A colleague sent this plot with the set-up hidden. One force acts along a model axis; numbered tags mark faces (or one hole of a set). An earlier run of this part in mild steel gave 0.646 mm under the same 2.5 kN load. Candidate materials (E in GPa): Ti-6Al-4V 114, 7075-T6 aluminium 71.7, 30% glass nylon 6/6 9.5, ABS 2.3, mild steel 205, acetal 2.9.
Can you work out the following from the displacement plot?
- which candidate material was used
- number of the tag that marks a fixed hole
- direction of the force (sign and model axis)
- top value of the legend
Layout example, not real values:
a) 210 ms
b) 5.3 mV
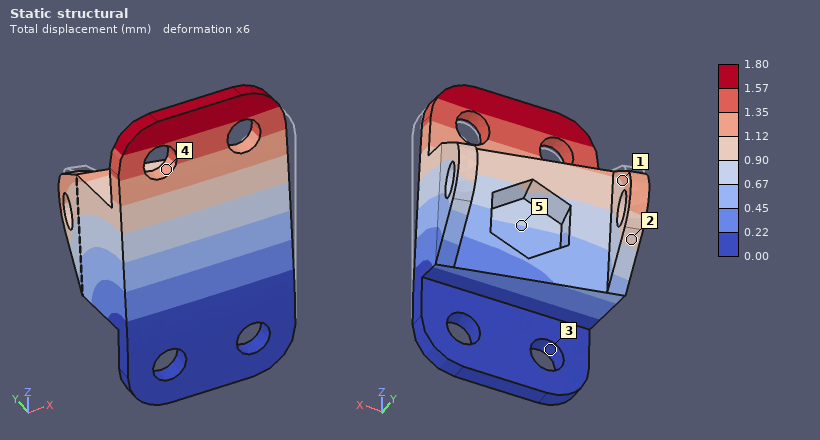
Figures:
a) 7075-T6 aluminium
b) 3
c) +Y
d) 1.80 mm
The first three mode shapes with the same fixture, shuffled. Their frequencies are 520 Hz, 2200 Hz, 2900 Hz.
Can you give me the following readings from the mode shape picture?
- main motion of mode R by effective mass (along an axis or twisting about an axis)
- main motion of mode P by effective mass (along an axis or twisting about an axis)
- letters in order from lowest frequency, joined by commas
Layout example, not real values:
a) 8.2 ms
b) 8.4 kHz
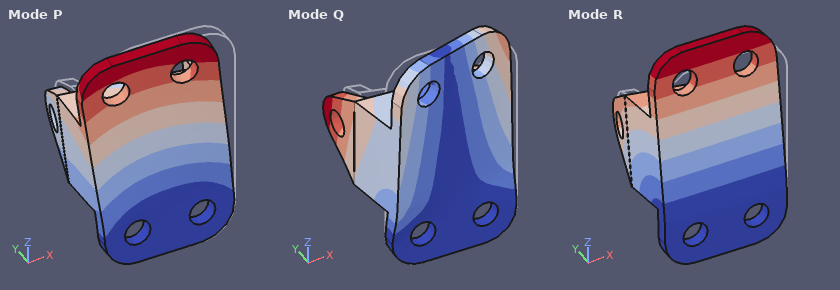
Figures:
a) along Y
b) along X
c) R, Q, P
